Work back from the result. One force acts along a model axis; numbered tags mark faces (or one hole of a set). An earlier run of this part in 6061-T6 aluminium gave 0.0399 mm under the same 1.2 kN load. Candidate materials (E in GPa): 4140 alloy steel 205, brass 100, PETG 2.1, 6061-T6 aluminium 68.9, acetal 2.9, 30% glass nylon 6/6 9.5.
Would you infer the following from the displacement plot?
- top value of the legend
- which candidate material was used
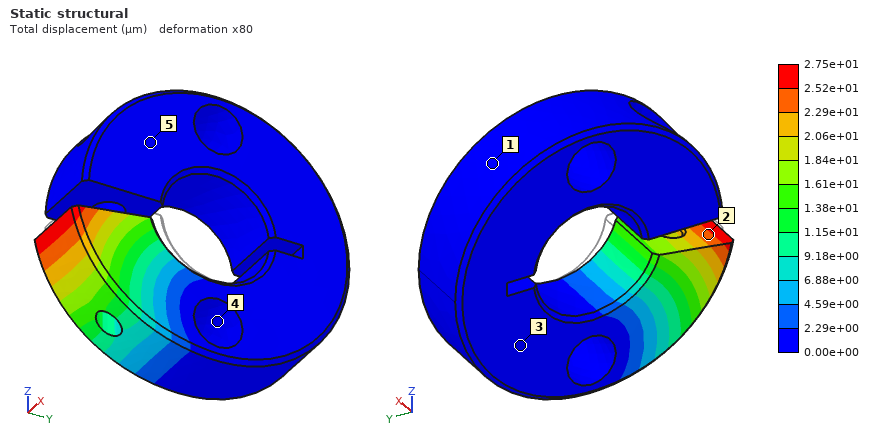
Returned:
2.75e+01 µm
brass
